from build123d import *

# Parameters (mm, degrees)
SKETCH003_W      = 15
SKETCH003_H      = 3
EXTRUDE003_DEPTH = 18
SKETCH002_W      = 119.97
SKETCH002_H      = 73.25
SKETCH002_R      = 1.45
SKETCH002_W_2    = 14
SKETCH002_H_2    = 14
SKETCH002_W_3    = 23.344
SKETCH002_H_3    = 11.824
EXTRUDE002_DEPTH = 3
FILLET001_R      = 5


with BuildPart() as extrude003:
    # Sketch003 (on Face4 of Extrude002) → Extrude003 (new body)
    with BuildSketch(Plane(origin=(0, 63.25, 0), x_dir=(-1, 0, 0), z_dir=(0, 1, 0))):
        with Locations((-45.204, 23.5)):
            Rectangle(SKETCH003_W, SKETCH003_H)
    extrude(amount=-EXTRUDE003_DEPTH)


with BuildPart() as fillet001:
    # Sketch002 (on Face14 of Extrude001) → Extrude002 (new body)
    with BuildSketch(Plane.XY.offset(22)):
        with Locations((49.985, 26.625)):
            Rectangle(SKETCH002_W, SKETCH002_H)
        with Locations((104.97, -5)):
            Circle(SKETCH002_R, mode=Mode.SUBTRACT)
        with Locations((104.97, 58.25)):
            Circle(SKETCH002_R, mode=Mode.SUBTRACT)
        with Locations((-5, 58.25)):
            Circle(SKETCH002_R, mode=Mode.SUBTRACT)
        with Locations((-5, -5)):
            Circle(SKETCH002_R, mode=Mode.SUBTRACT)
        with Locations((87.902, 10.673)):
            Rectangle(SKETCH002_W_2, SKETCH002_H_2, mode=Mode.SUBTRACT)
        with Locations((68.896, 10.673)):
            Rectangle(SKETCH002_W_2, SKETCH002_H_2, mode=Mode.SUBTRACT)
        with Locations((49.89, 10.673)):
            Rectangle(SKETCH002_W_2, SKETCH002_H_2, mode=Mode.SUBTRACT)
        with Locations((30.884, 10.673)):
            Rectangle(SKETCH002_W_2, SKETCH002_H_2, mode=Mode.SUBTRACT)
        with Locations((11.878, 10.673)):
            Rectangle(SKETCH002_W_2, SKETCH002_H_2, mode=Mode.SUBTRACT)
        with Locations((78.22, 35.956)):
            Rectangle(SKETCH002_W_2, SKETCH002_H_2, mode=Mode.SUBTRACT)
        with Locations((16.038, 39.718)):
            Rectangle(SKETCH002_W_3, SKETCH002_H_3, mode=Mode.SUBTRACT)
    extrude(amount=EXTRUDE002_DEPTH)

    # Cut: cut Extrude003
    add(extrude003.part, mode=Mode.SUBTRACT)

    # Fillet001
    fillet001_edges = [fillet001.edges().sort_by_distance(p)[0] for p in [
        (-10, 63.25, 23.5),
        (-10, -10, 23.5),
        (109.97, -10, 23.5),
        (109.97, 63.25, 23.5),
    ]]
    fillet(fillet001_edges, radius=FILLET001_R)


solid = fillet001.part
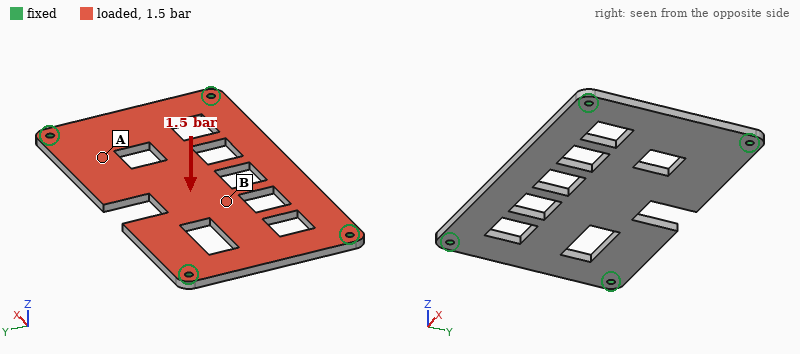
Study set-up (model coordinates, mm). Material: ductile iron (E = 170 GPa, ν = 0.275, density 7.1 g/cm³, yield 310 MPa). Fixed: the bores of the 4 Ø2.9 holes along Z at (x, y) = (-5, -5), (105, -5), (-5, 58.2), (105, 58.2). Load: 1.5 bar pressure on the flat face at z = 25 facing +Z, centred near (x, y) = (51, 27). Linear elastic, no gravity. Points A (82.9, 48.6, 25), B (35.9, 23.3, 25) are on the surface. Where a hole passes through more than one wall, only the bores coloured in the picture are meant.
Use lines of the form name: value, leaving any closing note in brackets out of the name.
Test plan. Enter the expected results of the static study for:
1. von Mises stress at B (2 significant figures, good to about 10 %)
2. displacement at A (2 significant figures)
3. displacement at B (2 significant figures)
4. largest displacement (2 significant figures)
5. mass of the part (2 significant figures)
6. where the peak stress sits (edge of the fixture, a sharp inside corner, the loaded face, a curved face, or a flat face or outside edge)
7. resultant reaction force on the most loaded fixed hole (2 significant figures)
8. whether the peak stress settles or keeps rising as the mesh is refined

von Mises stress at B: 48 MPa
displacement at A: 0.11 mm
displacement at B: 0.23 mm
largest displacement: 0.25 mm
mass of the part: 150 g
where the peak stress sits: edge of the fixture
resultant reaction force on the most loaded fixed hole: 280 N
whether the peak stress settles or keeps rising as the mesh is refined: keeps rising
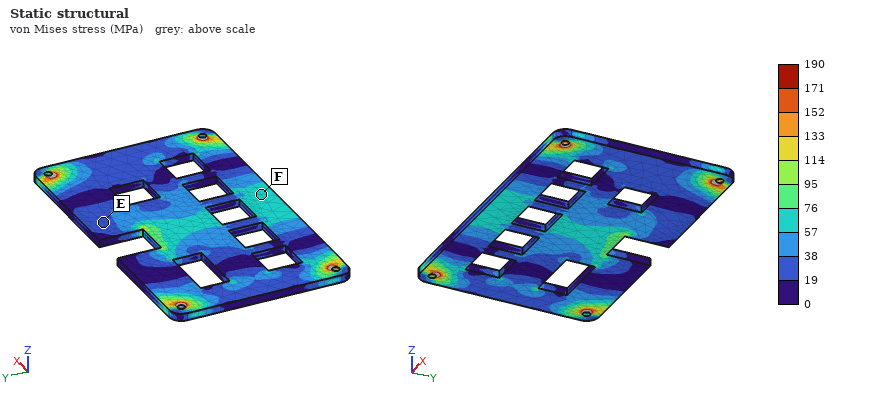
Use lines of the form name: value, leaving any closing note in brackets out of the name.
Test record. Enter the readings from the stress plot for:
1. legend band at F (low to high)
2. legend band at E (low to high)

legend band at F: 57 to 76 MPa
legend band at E: 19 to 38 MPa
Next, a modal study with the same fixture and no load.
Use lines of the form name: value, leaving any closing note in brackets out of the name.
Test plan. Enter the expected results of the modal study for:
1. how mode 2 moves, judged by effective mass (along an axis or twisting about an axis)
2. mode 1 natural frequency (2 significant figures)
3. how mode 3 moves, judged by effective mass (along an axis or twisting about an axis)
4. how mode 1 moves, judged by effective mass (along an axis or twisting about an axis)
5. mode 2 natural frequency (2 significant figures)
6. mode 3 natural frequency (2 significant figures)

how mode 2 moves, judged by effective mass: twisting about X
mode 1 natural frequency: 980 Hz
how mode 3 moves, judged by effective mass: twisting about Y
how mode 1 moves, judged by effective mass: along Z
mode 2 natural frequency: 1600 Hz
mode 3 natural frequency: 2500 Hz
